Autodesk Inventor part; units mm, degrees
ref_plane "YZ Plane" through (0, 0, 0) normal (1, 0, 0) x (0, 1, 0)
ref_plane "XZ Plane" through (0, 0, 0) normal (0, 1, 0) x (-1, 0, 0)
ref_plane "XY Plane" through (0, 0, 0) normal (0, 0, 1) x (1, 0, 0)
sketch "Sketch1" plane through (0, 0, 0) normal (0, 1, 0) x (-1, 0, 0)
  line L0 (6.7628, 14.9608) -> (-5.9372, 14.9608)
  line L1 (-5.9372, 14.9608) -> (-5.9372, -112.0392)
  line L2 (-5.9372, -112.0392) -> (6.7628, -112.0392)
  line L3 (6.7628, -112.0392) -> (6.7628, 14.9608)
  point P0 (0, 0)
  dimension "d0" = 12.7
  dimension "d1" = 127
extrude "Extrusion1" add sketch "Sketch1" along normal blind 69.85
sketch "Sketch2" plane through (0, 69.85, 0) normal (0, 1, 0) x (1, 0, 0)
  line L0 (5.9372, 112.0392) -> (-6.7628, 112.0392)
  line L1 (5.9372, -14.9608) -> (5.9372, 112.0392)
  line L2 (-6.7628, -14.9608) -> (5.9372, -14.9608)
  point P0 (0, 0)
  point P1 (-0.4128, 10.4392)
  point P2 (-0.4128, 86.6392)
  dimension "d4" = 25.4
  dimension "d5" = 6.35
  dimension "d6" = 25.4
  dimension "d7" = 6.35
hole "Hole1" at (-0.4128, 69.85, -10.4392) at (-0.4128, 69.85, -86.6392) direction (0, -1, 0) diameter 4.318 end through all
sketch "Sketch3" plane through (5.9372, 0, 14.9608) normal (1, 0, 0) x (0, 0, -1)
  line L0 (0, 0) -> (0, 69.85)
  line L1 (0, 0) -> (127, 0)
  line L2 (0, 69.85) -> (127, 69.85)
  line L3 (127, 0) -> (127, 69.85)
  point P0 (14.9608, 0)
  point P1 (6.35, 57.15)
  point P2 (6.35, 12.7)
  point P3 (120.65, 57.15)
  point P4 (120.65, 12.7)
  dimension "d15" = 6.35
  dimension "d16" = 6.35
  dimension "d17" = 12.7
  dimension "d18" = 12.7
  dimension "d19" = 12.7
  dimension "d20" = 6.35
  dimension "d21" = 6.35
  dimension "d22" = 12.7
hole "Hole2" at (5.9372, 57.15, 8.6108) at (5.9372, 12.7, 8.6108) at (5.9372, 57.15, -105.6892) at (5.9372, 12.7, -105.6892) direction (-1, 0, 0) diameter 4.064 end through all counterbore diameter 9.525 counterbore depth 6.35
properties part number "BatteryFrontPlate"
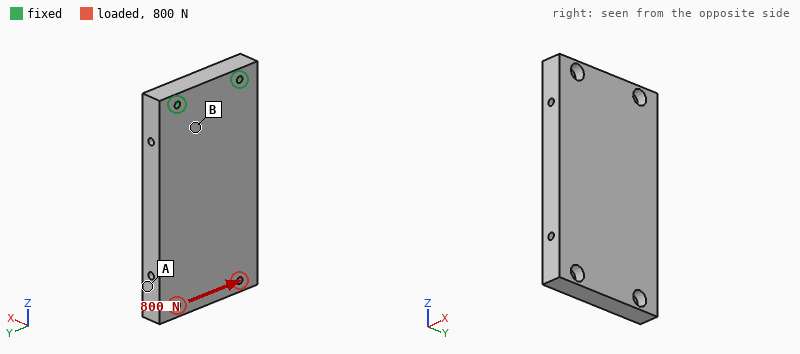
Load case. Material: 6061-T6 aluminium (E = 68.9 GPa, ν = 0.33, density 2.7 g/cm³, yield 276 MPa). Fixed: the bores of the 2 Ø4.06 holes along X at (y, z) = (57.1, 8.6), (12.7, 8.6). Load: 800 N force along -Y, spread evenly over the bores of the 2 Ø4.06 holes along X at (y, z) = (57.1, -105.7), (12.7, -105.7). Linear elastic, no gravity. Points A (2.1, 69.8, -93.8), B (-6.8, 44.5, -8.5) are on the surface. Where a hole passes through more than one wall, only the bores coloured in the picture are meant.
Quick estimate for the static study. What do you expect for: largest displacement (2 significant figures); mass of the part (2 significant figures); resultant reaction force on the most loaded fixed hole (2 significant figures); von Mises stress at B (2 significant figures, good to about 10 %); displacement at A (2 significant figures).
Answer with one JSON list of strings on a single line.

["46 µm", "290 g", "2.0 kN", "8.5 MPa", "36 µm"]
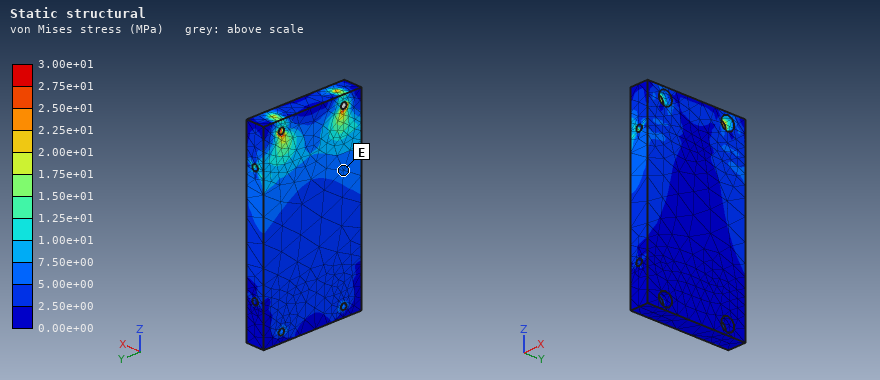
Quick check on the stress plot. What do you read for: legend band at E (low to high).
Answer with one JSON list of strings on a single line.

["5.00e+00 to 7.50e+00 MPa"]
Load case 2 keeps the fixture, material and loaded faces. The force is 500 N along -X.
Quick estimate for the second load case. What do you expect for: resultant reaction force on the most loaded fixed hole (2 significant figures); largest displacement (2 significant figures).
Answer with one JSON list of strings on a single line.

["290 N", "0.73 mm"]
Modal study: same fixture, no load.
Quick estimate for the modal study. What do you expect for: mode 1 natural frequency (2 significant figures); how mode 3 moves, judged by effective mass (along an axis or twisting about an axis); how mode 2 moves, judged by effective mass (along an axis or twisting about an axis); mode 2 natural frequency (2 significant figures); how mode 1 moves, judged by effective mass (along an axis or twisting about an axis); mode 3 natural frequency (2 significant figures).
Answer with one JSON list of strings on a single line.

["450 Hz", "along Y", "along Y", "2200 Hz", "along X", "2500 Hz"]
